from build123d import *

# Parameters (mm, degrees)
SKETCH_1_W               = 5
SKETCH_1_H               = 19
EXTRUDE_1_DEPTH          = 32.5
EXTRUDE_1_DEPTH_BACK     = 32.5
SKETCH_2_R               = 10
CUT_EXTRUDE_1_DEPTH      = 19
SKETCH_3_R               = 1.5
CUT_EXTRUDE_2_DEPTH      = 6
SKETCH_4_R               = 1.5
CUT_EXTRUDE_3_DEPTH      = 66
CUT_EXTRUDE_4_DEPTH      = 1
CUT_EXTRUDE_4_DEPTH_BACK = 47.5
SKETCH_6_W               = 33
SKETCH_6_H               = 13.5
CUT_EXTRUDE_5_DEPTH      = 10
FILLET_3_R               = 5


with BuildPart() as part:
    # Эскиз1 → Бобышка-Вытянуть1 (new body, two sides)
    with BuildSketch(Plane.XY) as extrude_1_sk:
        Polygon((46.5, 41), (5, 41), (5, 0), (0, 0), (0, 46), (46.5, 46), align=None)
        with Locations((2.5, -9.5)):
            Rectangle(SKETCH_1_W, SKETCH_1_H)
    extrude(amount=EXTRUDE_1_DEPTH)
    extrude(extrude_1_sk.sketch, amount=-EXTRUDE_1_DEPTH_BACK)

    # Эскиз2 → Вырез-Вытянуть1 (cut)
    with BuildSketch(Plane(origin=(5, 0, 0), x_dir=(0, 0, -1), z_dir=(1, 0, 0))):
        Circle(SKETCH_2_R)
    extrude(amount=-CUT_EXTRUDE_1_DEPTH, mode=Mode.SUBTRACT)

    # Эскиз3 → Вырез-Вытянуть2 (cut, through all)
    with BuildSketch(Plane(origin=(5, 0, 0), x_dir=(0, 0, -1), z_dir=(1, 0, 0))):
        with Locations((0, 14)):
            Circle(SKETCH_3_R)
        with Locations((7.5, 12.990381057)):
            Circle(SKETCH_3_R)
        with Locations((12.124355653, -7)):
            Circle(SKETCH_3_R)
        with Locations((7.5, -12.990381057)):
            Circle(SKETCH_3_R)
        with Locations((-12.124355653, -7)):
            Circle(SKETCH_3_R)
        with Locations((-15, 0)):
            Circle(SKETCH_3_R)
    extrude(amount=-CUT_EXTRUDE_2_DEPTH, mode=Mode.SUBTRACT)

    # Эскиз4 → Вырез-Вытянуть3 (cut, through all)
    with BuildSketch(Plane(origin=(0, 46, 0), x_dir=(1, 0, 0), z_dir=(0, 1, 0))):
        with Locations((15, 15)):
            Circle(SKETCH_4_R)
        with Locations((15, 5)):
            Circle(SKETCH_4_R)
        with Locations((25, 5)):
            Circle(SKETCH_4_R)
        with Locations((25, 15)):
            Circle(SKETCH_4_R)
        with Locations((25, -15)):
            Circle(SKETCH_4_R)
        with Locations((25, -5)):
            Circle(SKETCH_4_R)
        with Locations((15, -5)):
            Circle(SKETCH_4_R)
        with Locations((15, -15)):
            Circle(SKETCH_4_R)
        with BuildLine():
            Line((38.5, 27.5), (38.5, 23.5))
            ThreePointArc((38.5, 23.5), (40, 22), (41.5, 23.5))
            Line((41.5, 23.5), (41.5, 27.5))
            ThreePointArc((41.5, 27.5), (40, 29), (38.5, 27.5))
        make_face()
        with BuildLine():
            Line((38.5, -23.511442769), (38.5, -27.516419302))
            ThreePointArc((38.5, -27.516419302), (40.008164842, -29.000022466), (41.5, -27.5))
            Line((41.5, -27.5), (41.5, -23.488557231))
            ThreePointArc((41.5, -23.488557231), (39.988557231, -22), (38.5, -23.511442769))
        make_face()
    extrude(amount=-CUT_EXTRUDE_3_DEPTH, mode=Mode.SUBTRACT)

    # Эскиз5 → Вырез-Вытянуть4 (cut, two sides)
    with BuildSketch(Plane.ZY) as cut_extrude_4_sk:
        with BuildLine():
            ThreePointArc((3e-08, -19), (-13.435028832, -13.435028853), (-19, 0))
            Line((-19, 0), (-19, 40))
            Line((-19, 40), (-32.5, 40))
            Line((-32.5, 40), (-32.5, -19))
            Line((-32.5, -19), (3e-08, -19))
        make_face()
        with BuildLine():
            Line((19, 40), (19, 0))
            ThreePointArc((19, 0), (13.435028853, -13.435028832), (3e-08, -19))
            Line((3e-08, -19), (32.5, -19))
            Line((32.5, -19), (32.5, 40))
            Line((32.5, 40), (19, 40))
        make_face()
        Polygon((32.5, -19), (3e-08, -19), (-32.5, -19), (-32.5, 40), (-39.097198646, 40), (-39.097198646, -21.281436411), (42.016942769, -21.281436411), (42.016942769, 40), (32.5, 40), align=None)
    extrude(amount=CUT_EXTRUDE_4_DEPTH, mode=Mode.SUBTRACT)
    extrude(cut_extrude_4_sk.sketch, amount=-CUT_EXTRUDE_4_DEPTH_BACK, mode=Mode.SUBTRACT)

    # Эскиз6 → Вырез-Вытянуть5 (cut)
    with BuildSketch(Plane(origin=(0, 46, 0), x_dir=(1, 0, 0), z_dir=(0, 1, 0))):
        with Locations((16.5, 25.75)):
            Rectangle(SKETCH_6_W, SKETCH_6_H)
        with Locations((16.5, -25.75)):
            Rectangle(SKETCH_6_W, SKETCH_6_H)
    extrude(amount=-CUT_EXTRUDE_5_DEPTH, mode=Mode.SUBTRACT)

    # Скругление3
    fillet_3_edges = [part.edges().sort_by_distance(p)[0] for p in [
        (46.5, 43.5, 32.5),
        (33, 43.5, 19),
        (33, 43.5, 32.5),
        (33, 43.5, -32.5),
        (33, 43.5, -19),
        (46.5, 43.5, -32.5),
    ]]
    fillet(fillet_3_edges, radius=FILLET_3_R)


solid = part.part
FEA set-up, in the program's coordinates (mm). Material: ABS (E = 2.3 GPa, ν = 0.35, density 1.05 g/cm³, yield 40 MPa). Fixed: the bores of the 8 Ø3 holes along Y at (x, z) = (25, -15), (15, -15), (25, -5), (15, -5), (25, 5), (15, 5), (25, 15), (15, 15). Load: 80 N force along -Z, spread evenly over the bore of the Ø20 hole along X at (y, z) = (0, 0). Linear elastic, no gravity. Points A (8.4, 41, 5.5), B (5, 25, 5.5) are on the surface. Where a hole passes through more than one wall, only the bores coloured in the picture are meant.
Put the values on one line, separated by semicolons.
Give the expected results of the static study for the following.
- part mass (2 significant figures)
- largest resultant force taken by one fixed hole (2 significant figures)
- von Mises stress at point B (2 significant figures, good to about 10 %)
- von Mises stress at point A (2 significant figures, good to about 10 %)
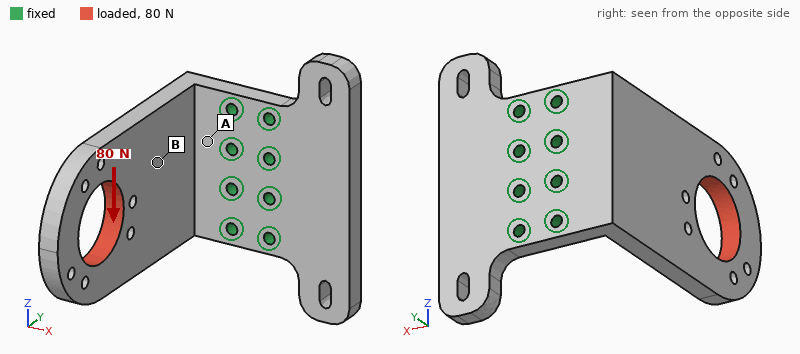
20 g; 110 N; 2.1 MPa; 6.1 MPa
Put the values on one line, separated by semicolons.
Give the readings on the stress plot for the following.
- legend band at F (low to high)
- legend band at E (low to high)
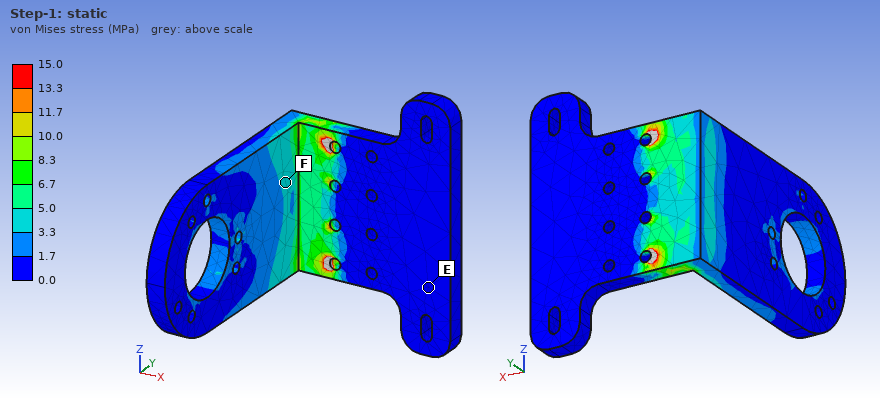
3.3 to 5.0 MPa; 0.0 to 1.7 MPa
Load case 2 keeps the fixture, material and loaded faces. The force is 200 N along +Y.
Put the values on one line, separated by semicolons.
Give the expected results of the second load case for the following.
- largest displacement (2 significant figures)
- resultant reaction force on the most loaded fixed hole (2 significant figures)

1.0 mm; 66 N
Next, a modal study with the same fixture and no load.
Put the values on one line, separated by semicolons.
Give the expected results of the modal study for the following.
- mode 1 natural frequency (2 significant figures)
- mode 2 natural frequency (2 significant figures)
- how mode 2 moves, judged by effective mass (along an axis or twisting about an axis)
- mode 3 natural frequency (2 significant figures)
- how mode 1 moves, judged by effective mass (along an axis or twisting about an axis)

310 Hz; 850 Hz; along Z; 1200 Hz; along X
